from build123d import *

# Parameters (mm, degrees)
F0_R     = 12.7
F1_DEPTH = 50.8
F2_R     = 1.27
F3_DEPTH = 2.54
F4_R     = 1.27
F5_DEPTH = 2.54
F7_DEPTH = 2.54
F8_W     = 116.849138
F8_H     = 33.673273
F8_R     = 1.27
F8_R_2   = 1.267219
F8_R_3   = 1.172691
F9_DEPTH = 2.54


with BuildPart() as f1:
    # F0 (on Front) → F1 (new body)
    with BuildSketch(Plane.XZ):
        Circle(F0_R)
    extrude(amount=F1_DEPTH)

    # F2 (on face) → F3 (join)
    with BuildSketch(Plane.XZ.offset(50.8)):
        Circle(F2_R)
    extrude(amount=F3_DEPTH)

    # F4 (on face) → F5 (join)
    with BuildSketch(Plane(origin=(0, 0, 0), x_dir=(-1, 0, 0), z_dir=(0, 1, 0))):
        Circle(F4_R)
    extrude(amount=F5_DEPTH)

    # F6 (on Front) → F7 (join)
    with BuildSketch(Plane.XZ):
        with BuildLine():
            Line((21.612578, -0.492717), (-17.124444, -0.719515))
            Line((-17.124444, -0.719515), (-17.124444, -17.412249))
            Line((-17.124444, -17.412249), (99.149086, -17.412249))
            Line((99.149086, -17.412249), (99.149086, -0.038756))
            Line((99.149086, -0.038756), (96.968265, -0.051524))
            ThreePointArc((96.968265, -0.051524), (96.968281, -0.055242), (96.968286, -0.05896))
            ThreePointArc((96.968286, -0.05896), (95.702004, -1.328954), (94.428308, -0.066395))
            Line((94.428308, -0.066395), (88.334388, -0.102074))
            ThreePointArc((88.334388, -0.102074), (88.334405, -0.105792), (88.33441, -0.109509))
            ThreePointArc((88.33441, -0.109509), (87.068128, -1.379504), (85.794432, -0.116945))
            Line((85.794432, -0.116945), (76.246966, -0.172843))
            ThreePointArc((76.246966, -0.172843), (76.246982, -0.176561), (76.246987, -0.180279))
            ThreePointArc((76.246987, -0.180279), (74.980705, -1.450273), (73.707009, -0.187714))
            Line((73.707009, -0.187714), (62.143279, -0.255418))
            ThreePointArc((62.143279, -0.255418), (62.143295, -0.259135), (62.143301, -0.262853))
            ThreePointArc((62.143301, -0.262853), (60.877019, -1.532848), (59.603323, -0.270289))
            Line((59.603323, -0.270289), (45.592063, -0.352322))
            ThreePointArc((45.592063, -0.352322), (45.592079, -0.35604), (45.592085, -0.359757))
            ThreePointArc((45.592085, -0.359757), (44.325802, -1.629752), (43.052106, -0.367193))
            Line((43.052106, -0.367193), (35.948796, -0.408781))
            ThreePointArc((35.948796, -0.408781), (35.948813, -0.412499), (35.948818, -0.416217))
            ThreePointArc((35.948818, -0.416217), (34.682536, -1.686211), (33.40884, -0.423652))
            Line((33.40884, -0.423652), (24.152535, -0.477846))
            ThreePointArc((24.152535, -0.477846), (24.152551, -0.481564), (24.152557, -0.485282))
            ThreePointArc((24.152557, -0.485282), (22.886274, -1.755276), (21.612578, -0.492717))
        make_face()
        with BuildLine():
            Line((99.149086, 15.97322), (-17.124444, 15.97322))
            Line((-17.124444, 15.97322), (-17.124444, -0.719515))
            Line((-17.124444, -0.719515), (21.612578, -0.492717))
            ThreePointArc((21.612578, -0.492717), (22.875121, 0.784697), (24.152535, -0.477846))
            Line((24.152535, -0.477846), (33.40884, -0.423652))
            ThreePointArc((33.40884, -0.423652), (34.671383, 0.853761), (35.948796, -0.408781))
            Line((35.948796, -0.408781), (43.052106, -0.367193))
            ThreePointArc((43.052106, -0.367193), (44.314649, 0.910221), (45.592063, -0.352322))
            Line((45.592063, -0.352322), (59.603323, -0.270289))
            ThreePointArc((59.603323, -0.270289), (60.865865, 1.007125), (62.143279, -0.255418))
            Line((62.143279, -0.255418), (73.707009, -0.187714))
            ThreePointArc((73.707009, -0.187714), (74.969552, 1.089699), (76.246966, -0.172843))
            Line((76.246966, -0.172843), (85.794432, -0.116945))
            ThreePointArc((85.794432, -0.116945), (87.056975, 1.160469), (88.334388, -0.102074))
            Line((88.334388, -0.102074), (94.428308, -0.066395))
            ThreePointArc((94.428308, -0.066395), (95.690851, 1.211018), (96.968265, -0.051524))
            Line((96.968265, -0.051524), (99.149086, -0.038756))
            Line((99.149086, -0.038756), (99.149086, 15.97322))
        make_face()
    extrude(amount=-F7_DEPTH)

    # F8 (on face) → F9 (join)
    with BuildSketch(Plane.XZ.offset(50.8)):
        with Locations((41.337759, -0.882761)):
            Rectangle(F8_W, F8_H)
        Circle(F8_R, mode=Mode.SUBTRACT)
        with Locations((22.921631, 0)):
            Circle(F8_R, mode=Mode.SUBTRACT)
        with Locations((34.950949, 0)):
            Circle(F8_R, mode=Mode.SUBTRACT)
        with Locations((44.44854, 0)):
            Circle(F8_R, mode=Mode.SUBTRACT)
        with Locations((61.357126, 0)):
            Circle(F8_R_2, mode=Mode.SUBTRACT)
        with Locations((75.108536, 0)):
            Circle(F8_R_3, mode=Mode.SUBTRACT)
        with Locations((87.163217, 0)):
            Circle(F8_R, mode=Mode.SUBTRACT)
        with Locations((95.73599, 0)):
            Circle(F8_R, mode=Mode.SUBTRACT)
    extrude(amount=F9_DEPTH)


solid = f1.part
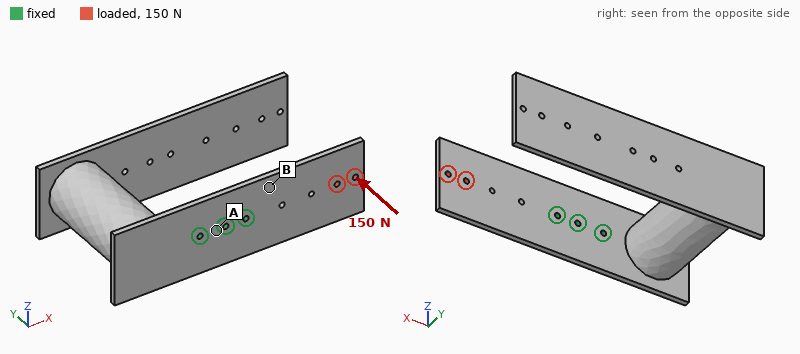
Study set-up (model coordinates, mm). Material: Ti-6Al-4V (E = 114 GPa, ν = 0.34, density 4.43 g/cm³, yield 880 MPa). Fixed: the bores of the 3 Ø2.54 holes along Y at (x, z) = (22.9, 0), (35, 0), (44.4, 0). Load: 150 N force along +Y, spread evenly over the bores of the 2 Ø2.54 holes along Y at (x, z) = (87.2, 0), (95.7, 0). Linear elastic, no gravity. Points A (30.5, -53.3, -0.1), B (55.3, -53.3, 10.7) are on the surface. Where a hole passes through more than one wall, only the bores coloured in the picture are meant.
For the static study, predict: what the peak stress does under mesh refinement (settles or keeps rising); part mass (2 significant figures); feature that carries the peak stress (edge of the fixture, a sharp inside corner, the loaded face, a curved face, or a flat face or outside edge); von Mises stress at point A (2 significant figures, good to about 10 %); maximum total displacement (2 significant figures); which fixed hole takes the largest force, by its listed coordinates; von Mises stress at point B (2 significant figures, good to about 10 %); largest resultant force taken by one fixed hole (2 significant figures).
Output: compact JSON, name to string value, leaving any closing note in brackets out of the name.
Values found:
{"what the peak stress does under mesh refinement": "keeps rising", "part mass": "200 g", "feature that carries the peak stress": "edge of the fixture", "von Mises stress at point A": "33 MPa", "maximum total displacement": "1.4 mm", "which fixed hole takes the largest force, by its listed coordinates": "(44.4, 0)", "von Mises stress at point B": "150 MPa", "largest resultant force taken by one fixed hole": "510 N"}
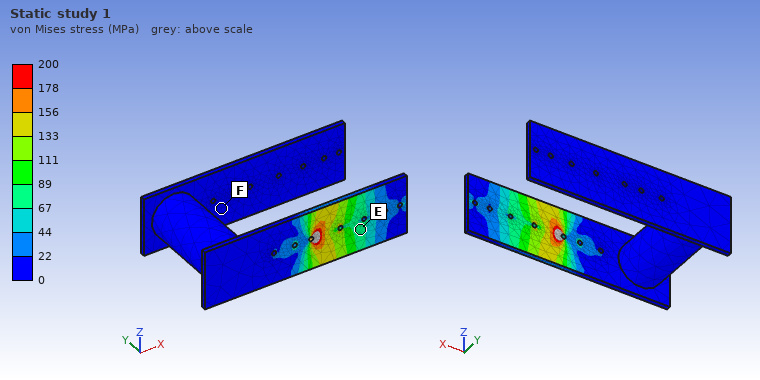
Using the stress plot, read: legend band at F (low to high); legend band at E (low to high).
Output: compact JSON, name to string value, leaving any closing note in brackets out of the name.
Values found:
{"legend band at F": "0 to 22 MPa", "legend band at E": "67 to 89 MPa"}
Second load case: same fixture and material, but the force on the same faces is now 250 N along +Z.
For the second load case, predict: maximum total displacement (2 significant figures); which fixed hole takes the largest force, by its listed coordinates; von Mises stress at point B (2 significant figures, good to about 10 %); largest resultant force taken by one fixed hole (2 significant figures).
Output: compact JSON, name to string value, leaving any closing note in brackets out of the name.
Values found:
{"maximum total displacement": "35 µm", "which fixed hole takes the largest force, by its listed coordinates": "(44.4, 0)", "von Mises stress at point B": "14 MPa", "largest resultant force taken by one fixed hole": "770 N"}
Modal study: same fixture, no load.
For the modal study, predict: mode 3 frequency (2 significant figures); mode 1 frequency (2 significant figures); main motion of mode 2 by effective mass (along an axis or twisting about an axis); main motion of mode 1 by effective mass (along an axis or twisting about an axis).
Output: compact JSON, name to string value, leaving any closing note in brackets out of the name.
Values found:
{"mode 3 frequency": "310 Hz", "mode 1 frequency": "160 Hz", "main motion of mode 2 by effective mass": "along Z", "main motion of mode 1 by effective mass": "along X"}
